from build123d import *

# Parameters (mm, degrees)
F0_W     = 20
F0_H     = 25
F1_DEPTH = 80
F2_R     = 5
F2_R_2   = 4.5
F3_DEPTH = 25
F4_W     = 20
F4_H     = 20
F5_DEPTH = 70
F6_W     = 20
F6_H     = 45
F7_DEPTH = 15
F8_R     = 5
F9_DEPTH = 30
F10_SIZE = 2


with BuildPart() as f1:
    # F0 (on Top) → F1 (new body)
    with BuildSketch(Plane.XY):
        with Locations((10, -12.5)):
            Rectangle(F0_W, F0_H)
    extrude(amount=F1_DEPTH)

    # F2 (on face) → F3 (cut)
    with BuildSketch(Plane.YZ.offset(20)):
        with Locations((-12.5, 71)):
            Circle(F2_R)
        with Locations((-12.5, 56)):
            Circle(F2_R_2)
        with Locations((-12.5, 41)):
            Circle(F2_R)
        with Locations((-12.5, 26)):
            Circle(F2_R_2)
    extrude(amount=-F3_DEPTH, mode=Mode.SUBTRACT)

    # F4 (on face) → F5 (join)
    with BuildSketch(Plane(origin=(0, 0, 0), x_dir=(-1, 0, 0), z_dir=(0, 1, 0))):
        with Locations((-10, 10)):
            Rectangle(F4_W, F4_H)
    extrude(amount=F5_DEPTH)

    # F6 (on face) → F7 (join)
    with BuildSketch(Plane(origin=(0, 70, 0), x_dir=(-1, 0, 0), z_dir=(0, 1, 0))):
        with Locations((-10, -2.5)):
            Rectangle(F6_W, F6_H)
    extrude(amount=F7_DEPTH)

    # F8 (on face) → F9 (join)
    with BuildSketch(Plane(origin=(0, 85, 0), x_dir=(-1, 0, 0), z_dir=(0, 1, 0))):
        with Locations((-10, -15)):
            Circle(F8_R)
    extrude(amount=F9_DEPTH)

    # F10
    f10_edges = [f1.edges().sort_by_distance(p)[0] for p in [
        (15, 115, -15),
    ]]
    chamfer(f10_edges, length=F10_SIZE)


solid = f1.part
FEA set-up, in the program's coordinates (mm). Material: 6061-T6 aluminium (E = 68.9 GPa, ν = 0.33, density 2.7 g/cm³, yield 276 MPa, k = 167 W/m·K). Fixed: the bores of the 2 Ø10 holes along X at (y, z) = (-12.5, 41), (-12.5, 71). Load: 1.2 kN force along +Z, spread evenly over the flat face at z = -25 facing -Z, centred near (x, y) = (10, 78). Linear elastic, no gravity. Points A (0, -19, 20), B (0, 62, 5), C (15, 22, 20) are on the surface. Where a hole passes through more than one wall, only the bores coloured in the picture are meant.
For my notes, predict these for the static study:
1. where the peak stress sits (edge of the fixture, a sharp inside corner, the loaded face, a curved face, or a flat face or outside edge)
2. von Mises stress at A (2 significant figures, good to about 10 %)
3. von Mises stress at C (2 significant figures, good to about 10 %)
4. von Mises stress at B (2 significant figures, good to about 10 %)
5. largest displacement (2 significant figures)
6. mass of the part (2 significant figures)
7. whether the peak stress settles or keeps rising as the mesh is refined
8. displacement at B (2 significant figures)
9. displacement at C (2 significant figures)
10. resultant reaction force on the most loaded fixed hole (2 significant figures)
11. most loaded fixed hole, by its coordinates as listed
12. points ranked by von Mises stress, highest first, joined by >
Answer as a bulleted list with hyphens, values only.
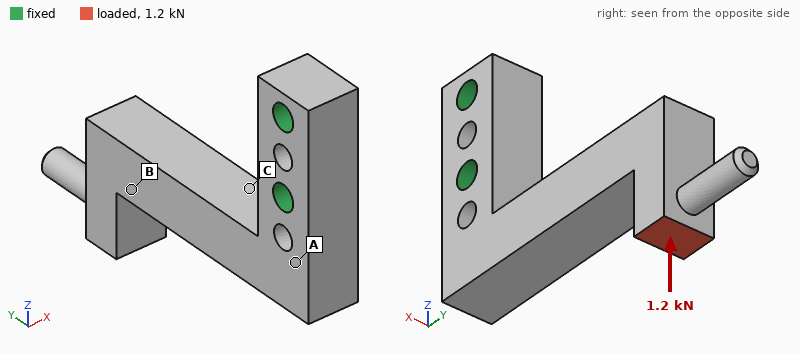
- a sharp inside corner
- 30 MPa
- 49 MPa
- 9.4 MPa
- 0.76 mm
- 210 g
- keeps rising
- 0.37 mm
- 0.12 mm
- 1.5 kN
- (-12.5, 41)
- C > A > B
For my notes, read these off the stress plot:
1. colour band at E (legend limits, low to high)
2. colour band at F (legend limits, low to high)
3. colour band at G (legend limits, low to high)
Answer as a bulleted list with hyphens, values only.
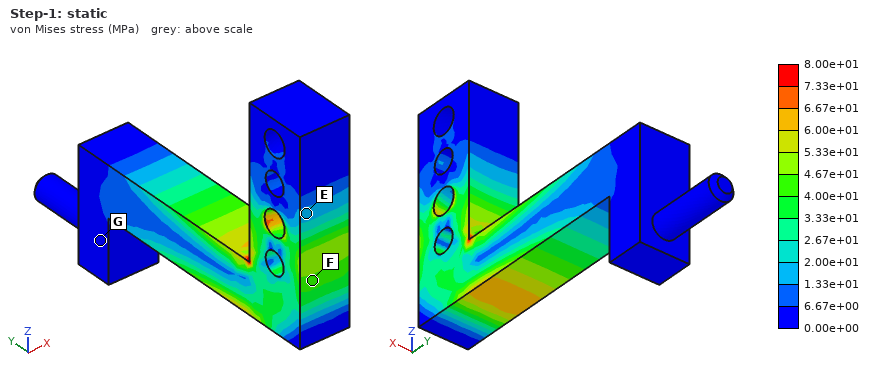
- 1.33e+01 to 2.00e+01 MPa
- 4.00e+01 to 4.67e+01 MPa
- 0.00e+00 to 6.67e+00 MPa
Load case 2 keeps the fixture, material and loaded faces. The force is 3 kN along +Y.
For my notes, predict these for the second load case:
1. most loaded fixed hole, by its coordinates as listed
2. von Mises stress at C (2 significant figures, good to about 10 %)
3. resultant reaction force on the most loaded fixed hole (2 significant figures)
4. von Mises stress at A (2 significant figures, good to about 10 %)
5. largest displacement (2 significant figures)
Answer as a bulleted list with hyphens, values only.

- (-12.5, 41)
- 71 MPa
- 4.7 kN
- 45 MPa
- 1.4 mm
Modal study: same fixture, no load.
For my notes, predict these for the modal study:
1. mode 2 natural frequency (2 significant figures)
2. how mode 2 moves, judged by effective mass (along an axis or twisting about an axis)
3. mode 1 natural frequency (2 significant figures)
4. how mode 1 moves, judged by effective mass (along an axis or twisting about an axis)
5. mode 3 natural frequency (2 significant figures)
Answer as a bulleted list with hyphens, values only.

- 950 Hz
- along Z
- 820 Hz
- along X
- 3500 Hz
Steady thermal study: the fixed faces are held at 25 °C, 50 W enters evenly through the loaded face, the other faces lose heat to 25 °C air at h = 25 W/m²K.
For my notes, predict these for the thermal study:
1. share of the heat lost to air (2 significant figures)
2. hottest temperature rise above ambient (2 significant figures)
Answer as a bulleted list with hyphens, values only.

- 27 %
- 89 K
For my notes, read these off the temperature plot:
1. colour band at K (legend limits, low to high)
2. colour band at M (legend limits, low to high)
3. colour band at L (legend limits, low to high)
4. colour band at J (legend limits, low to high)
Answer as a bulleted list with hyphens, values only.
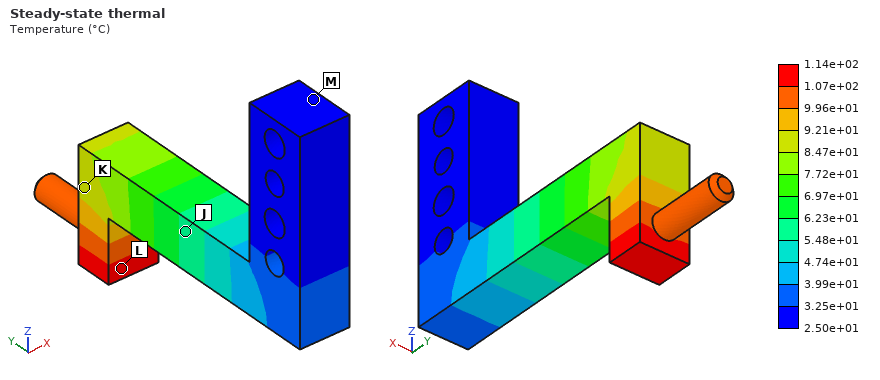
- 8.47e+01 to 9.21e+01 °C
- 2.50e+01 to 3.25e+01 °C
- 1.07e+02 to 1.14e+02 °C
- 5.48e+01 to 6.23e+01 °C
